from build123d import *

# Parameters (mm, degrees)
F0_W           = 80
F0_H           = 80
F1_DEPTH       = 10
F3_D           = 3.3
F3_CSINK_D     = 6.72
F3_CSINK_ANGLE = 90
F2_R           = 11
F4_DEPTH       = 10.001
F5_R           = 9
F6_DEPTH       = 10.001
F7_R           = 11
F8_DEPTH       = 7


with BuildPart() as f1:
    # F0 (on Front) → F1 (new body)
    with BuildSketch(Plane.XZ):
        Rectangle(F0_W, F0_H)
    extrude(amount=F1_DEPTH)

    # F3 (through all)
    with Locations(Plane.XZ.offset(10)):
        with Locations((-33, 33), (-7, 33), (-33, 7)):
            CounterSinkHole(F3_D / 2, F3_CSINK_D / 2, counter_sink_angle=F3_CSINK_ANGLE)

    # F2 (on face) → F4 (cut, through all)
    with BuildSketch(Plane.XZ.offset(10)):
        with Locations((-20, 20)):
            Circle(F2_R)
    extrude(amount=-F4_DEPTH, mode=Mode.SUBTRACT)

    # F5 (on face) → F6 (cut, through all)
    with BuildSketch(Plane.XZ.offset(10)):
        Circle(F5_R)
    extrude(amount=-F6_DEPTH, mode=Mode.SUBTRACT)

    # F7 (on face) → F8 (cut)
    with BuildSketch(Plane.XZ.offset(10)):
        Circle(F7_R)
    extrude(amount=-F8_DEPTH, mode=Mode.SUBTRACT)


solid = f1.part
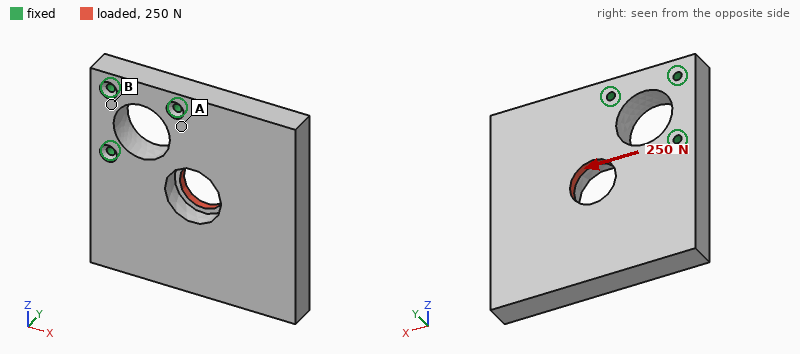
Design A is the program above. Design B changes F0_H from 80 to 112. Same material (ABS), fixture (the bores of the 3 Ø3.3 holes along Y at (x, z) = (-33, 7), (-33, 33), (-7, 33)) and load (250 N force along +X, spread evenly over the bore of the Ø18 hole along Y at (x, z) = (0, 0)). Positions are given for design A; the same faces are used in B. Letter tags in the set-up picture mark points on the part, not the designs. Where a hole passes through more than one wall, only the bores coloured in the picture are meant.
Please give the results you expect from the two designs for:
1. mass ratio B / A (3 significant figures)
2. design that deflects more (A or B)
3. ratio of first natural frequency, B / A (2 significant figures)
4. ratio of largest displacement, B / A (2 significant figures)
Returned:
1.45
A
0.78
0.87
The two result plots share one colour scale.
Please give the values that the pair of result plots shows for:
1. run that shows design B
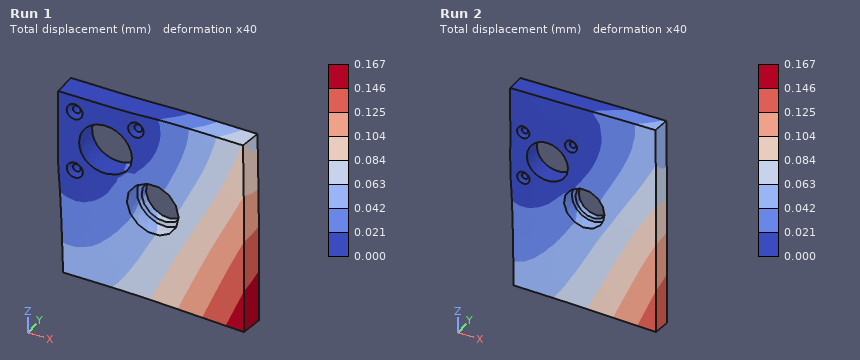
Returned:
Run 2
